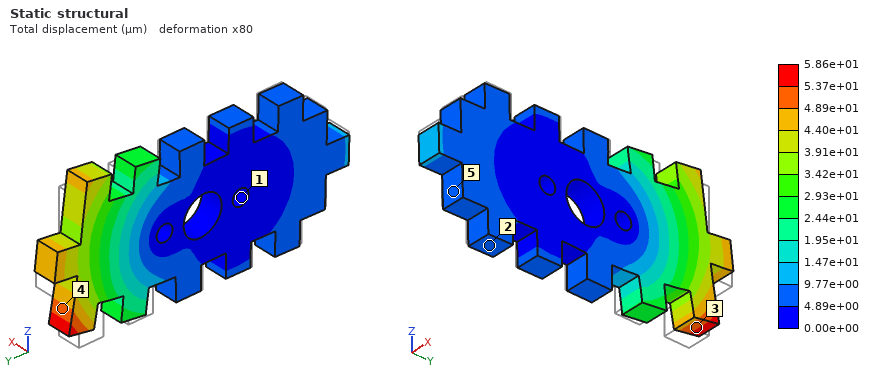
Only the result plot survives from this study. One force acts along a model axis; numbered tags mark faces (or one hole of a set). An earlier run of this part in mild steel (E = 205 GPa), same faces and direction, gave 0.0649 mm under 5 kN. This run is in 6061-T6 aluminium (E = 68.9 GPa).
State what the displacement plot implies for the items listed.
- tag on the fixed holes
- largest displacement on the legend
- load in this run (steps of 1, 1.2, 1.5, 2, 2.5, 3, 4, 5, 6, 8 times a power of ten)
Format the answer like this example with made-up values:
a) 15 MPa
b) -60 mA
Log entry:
a) 1
b) 5.86e+01 µm
c) 1.5 kN
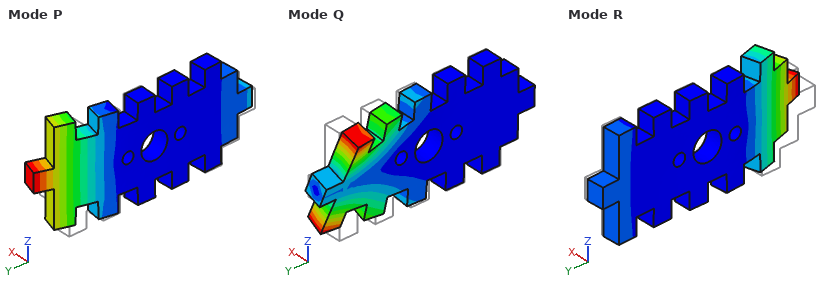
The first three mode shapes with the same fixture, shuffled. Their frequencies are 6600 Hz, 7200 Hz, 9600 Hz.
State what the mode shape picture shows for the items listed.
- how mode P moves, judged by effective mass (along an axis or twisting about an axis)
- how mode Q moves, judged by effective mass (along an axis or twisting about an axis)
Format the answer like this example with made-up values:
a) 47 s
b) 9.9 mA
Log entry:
a) along X
b) twisting about Y
